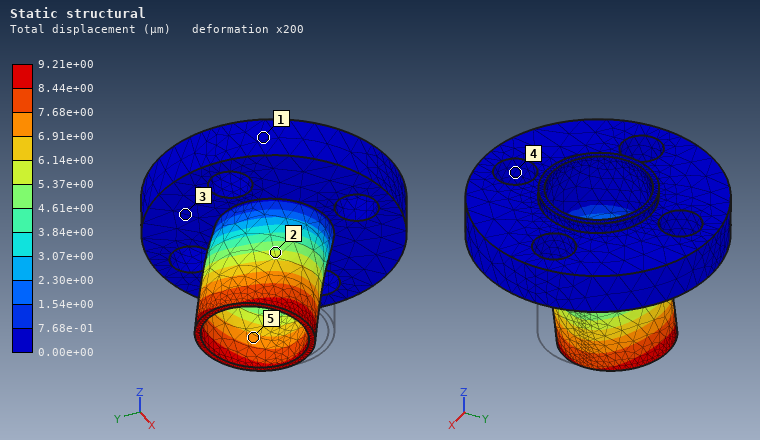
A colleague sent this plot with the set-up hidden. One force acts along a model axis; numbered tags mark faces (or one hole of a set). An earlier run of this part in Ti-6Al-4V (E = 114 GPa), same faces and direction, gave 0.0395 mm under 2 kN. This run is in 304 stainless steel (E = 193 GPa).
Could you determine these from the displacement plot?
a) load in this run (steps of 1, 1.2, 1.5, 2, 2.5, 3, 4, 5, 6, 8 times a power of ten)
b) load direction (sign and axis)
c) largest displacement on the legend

800 N
+Y
9.21e+00 µm
